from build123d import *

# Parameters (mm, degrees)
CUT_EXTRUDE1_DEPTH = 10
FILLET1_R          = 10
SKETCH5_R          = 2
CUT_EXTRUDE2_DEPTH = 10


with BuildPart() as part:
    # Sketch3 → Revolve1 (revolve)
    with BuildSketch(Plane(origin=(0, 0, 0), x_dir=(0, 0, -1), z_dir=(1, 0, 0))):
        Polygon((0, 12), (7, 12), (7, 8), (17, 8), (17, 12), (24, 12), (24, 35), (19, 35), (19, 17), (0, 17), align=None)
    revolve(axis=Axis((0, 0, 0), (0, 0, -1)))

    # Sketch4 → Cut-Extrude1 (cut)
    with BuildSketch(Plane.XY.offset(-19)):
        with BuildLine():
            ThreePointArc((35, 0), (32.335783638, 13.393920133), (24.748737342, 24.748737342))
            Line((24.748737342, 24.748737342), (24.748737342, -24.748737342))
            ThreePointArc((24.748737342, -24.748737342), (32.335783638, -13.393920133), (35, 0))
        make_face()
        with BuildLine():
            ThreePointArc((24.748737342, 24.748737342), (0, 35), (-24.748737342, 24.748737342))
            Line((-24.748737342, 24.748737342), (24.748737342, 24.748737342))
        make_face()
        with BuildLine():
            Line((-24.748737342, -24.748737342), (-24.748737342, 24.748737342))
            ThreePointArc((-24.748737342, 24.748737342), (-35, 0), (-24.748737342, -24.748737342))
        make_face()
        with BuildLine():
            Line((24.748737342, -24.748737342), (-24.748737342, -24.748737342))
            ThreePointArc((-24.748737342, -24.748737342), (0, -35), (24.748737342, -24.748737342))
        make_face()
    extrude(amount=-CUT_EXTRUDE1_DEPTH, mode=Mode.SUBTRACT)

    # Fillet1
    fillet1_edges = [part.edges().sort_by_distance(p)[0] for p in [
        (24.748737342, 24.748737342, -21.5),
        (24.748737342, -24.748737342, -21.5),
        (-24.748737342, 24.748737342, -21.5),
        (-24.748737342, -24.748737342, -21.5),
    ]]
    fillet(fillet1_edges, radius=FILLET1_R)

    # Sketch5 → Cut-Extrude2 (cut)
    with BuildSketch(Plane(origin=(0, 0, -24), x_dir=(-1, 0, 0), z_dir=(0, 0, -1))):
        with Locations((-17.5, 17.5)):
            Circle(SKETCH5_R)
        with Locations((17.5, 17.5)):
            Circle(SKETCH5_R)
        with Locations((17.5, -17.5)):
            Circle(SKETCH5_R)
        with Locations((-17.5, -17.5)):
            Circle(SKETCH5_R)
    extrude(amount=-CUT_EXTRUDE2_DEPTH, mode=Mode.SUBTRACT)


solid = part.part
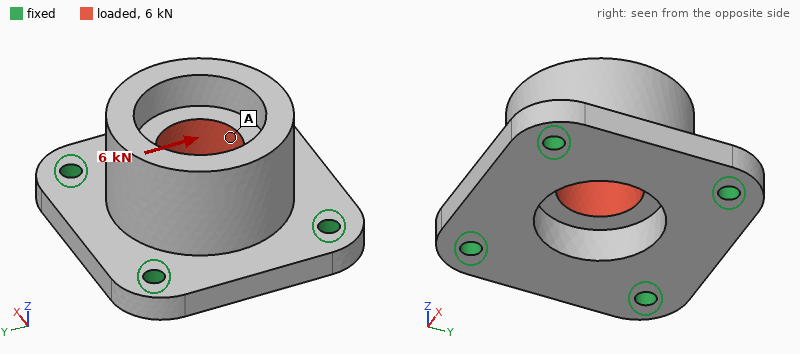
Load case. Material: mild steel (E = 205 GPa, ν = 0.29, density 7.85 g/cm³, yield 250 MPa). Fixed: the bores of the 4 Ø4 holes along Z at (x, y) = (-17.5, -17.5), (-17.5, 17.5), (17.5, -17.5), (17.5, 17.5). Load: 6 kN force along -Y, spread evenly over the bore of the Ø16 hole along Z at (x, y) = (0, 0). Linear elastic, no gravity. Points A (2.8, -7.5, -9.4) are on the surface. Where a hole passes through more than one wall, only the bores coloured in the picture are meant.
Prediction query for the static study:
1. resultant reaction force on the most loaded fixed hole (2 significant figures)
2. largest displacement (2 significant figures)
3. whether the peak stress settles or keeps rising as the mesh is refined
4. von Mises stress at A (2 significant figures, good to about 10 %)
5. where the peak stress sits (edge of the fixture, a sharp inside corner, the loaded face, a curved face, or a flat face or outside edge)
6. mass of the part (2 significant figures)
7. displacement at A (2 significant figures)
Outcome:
1.8 kN
9.0 µm
keeps rising
12 MPa
edge of the fixture
160 g
6.3 µm
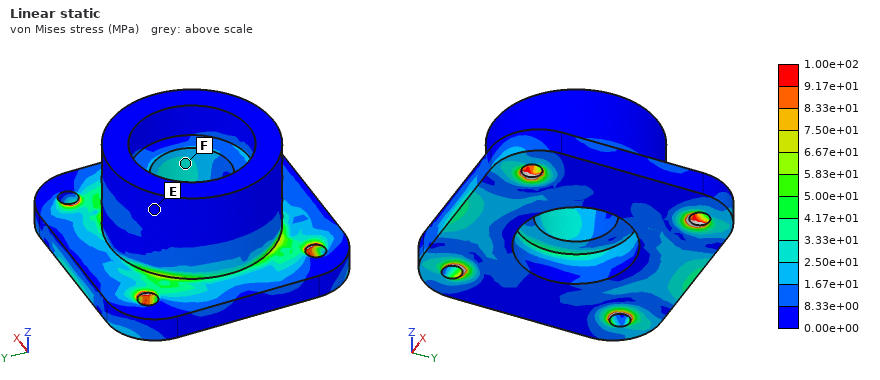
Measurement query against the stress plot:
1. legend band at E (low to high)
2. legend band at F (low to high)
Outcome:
0.00e+00 to 8.33e+00 MPa
2.50e+01 to 3.33e+01 MPa
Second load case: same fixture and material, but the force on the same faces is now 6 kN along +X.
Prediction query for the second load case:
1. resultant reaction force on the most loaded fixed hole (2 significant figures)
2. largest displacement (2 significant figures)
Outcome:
1.8 kN
9.0 µm
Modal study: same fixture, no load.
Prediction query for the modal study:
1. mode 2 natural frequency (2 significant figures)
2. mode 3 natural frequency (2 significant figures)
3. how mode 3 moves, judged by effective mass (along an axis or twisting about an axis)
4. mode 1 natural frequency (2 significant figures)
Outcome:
13 kHz
13 kHz
along Z
13 kHz
